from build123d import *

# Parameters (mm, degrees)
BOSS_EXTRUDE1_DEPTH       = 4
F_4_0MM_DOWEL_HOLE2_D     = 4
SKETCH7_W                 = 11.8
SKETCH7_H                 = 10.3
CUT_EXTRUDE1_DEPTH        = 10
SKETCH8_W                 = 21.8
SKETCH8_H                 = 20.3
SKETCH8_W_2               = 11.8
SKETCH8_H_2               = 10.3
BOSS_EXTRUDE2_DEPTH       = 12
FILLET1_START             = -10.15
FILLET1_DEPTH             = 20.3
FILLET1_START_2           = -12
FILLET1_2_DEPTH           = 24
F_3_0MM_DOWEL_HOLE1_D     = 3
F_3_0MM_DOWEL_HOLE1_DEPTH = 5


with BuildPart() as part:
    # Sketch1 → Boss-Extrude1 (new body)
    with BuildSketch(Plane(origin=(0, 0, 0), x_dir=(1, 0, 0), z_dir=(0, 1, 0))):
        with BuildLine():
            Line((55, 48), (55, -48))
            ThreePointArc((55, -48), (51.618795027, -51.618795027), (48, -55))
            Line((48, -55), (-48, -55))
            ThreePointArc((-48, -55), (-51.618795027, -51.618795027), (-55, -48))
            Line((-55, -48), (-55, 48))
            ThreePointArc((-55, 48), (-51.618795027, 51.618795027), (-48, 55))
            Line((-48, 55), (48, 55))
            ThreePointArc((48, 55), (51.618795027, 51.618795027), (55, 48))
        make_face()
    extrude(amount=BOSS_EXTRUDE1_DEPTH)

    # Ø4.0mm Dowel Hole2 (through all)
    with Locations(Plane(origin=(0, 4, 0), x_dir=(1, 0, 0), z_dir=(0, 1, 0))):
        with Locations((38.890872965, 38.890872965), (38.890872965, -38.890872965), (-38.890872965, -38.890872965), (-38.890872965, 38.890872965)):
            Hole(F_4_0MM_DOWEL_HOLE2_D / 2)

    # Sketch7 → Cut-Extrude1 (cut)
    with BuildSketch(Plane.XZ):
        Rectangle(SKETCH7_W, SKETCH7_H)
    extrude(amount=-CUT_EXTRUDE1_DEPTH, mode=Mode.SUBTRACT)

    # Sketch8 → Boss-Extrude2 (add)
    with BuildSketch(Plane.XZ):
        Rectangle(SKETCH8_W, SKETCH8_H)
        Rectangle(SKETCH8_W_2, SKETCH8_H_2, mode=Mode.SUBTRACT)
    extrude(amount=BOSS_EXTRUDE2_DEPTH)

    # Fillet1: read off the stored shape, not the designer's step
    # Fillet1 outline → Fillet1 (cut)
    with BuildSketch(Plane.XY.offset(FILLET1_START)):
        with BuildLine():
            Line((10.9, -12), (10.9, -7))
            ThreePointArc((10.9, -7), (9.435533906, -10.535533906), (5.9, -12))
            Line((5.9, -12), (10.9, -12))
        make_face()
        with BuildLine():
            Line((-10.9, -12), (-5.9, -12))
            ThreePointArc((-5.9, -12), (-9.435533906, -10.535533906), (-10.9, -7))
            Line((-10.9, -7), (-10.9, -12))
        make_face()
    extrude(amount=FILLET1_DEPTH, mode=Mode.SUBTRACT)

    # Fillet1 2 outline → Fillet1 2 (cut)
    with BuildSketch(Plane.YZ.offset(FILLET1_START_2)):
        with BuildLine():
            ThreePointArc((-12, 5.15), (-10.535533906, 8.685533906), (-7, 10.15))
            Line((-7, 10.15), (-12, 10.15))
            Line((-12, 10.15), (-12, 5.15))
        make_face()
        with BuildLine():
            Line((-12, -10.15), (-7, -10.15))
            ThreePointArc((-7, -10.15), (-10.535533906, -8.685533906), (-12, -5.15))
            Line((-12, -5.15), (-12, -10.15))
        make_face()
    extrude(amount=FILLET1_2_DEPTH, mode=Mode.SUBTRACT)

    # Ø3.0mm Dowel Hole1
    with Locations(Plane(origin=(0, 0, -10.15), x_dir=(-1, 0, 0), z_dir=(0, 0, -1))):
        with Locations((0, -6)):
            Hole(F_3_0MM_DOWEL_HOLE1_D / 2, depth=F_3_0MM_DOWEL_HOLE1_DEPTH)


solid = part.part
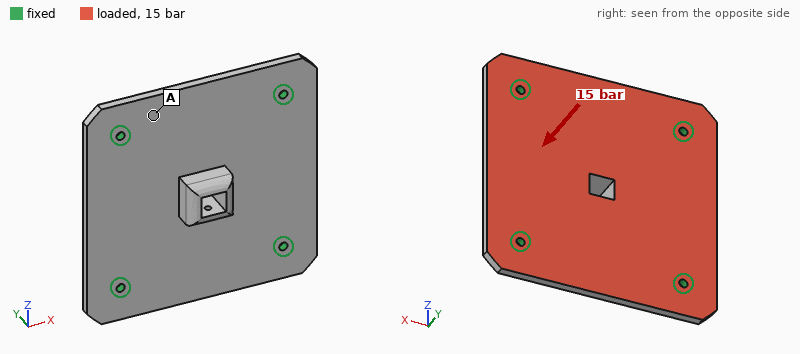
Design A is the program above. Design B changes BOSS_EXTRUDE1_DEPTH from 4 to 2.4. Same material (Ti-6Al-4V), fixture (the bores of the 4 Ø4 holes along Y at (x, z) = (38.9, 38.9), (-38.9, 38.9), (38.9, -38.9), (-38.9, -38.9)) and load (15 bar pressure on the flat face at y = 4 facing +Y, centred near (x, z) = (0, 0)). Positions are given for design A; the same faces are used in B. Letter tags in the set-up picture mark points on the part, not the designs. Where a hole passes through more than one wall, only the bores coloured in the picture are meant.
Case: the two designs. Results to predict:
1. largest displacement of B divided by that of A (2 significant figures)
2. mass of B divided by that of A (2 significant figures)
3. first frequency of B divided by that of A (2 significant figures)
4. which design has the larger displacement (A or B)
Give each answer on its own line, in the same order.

4.1
0.63
0.60
B
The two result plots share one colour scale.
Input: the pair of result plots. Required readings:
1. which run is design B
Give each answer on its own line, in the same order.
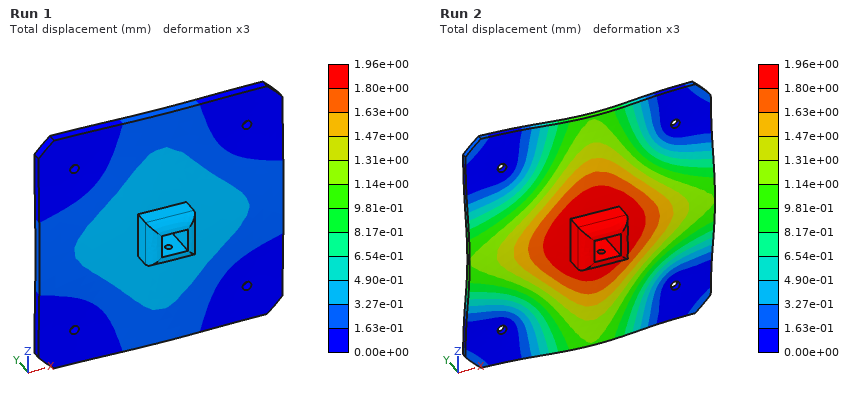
Run 2
